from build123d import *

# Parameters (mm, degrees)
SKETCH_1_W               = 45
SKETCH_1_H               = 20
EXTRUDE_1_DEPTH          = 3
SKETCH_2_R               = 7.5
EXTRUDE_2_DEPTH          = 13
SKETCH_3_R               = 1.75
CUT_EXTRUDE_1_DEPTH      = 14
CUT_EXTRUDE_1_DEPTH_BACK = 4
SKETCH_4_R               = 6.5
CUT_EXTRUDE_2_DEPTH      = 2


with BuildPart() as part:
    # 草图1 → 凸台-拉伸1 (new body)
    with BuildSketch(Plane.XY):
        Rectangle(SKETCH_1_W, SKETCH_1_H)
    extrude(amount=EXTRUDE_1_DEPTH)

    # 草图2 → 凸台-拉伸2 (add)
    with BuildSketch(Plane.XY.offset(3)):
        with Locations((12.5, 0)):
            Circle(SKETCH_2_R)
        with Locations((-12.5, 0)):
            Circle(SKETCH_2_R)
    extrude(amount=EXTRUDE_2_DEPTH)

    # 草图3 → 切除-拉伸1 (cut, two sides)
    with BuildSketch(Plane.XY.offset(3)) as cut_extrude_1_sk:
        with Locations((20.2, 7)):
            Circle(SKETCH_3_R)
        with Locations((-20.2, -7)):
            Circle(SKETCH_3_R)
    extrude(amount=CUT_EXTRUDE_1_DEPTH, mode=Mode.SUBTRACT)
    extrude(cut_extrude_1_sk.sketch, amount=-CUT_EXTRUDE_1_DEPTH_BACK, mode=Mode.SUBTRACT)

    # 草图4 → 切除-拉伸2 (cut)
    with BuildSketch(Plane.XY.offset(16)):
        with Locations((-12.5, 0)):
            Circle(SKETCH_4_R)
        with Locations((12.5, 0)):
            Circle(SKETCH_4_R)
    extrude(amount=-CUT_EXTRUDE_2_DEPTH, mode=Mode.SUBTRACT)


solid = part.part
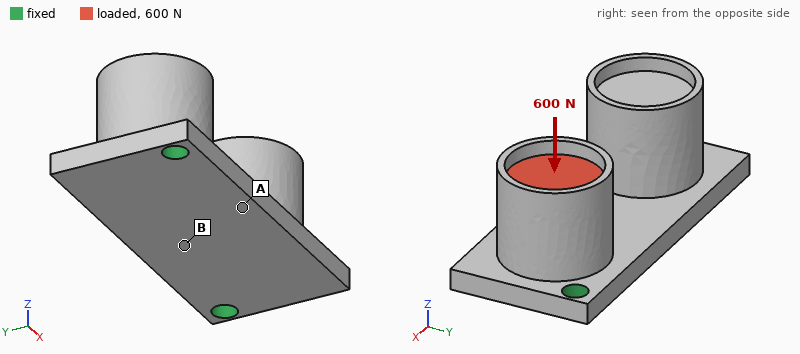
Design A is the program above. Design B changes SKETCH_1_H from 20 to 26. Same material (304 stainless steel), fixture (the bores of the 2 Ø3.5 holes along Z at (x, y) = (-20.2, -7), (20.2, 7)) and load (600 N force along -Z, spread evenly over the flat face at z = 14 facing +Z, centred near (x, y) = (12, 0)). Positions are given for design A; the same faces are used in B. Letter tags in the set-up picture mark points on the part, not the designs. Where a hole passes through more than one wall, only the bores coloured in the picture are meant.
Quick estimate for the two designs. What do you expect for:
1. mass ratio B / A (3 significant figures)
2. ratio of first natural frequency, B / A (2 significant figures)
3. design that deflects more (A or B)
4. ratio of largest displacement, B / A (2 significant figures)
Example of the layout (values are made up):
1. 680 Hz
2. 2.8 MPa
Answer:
1. 1.12
2. 1.0
3. A
4. 0.86
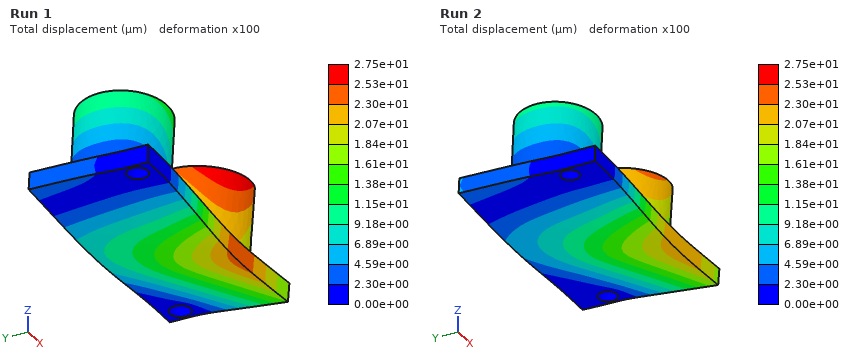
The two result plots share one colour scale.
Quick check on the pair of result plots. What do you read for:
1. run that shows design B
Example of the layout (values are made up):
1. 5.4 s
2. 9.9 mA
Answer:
1. Run 2
